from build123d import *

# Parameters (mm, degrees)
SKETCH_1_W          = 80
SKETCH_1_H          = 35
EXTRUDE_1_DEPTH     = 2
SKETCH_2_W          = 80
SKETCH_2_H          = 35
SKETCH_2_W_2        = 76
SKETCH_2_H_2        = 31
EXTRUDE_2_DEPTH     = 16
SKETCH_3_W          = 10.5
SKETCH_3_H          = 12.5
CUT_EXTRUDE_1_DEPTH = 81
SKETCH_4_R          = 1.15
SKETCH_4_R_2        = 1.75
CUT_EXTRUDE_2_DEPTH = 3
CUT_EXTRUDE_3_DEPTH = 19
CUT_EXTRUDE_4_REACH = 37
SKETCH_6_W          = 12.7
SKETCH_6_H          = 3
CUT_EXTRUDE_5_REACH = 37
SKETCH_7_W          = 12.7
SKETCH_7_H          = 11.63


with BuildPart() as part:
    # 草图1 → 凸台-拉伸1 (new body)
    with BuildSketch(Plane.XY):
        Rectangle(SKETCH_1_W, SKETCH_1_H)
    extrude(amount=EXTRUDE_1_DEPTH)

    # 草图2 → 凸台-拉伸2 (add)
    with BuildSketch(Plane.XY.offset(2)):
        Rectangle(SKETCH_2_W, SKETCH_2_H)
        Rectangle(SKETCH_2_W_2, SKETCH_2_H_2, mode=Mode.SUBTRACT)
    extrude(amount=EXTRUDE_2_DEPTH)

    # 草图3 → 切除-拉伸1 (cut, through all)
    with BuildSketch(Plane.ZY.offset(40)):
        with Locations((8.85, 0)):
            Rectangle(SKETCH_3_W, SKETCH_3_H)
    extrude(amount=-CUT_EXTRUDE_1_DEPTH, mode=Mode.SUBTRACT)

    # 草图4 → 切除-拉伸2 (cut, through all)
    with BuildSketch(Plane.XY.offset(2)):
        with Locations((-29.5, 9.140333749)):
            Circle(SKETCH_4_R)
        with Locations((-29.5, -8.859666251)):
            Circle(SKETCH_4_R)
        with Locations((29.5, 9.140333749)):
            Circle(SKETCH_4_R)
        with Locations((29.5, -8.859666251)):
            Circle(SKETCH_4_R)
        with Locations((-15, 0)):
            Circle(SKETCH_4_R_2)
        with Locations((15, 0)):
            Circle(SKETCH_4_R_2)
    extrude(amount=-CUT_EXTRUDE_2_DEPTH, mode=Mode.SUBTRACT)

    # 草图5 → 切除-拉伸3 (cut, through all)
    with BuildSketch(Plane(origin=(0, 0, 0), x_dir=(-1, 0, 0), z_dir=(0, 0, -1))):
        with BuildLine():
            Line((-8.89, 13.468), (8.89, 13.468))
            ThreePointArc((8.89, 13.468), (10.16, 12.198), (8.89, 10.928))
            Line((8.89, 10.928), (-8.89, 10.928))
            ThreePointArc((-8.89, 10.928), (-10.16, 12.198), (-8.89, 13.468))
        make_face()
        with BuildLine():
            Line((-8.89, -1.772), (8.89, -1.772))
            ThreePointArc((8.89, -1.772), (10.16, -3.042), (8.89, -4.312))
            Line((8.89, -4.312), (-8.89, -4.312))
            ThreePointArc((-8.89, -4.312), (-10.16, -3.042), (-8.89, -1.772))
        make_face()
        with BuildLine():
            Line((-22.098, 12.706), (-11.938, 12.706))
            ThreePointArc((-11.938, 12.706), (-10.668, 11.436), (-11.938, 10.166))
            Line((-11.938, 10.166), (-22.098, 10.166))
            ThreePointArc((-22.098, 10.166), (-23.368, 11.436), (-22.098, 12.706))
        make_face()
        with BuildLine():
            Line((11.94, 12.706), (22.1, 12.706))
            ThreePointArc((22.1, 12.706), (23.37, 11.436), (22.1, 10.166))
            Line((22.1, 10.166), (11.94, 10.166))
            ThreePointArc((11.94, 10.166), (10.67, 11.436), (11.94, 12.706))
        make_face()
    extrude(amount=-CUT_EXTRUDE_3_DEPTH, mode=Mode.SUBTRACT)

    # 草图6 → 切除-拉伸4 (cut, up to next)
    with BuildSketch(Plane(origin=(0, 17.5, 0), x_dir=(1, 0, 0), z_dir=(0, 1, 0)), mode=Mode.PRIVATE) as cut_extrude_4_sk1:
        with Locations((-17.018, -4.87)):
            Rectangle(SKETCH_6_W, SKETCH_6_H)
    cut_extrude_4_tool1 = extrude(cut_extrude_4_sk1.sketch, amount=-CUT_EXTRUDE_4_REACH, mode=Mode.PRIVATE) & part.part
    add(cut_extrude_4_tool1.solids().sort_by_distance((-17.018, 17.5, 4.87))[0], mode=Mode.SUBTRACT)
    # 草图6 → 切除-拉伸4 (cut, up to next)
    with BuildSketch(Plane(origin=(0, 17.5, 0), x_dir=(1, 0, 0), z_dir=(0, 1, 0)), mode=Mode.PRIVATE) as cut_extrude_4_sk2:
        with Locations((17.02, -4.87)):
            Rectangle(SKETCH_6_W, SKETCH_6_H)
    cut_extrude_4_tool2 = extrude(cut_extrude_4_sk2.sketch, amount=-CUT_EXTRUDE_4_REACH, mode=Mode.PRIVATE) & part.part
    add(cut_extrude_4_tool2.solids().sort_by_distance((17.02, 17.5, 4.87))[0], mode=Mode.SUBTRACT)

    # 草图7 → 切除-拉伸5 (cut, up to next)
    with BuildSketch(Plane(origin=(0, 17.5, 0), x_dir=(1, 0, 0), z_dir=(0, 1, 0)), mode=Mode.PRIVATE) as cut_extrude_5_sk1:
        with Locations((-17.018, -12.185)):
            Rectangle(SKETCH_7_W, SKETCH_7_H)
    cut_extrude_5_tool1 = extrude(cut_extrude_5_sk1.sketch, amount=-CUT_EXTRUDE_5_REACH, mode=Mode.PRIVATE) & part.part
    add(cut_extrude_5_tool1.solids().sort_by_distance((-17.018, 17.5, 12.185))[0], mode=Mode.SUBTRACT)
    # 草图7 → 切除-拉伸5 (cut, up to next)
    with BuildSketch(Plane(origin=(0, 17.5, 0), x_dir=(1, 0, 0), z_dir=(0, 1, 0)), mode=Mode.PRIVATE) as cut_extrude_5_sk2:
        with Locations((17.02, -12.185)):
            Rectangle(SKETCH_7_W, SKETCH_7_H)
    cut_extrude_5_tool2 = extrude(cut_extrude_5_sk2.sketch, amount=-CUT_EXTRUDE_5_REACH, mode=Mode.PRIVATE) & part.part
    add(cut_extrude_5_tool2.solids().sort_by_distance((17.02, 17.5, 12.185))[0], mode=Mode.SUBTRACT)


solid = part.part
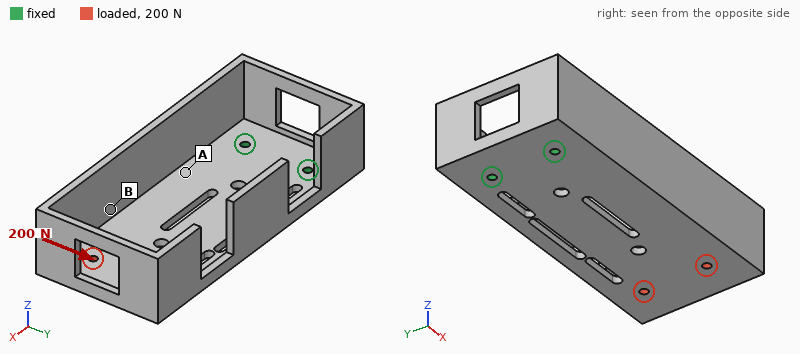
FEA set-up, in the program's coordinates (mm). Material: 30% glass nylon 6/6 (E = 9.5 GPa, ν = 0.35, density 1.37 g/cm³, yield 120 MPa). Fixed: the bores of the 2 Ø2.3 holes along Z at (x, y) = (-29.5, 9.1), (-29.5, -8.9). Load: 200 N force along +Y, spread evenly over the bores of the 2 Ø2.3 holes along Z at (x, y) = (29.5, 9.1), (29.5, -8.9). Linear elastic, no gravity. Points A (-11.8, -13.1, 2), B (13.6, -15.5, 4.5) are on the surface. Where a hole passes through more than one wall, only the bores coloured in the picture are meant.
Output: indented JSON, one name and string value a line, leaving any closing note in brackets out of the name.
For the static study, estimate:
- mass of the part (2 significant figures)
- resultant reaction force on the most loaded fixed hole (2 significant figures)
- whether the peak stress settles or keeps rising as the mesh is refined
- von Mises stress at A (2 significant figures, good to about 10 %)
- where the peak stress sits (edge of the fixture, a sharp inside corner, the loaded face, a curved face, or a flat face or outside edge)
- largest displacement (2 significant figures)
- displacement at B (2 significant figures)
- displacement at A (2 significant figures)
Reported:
{
  "mass of the part": "15 g",
  "resultant reaction force on the most loaded fixed hole": "630 N",
  "whether the peak stress settles or keeps rising as the mesh is refined": "keeps rising",
  "von Mises stress at A": "11 MPa",
  "where the peak stress sits": "edge of the fixture",
  "largest displacement": "0.53 mm",
  "displacement at B": "0.30 mm",
  "displacement at A": "0.097 mm"
}
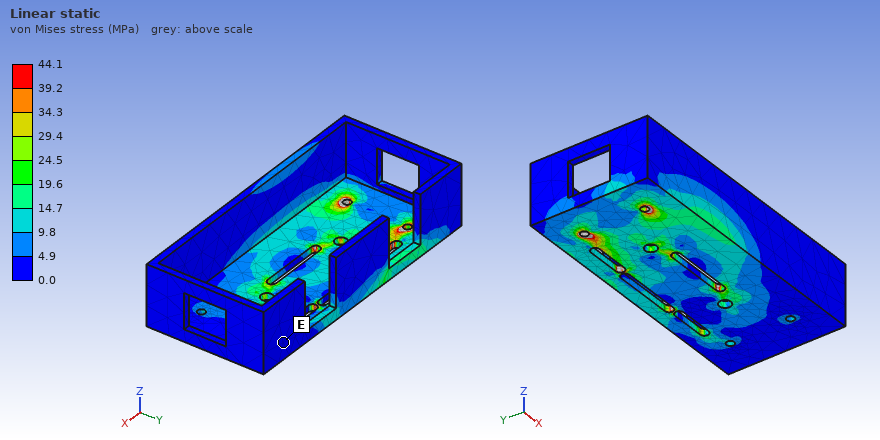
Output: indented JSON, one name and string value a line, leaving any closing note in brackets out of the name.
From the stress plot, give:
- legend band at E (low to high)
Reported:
{
  "legend band at E": "0.0 to 4.9 MPa"
}
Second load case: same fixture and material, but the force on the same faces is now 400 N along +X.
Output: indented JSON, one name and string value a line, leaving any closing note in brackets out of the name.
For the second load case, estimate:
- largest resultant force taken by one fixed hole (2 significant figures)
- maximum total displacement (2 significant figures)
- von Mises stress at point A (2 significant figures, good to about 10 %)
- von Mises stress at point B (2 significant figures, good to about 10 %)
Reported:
{
  "largest resultant force taken by one fixed hole": "200 N",
  "maximum total displacement": "0.13 mm",
  "von Mises stress at point A": "4.5 MPa",
  "von Mises stress at point B": "2.8 MPa"
}
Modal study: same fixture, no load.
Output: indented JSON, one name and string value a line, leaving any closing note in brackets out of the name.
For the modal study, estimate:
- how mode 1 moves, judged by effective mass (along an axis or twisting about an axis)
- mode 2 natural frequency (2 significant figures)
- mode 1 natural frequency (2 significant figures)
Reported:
{
  "how mode 1 moves, judged by effective mass": "along Z",
  "mode 2 natural frequency": "470 Hz",
  "mode 1 natural frequency": "230 Hz"
}
